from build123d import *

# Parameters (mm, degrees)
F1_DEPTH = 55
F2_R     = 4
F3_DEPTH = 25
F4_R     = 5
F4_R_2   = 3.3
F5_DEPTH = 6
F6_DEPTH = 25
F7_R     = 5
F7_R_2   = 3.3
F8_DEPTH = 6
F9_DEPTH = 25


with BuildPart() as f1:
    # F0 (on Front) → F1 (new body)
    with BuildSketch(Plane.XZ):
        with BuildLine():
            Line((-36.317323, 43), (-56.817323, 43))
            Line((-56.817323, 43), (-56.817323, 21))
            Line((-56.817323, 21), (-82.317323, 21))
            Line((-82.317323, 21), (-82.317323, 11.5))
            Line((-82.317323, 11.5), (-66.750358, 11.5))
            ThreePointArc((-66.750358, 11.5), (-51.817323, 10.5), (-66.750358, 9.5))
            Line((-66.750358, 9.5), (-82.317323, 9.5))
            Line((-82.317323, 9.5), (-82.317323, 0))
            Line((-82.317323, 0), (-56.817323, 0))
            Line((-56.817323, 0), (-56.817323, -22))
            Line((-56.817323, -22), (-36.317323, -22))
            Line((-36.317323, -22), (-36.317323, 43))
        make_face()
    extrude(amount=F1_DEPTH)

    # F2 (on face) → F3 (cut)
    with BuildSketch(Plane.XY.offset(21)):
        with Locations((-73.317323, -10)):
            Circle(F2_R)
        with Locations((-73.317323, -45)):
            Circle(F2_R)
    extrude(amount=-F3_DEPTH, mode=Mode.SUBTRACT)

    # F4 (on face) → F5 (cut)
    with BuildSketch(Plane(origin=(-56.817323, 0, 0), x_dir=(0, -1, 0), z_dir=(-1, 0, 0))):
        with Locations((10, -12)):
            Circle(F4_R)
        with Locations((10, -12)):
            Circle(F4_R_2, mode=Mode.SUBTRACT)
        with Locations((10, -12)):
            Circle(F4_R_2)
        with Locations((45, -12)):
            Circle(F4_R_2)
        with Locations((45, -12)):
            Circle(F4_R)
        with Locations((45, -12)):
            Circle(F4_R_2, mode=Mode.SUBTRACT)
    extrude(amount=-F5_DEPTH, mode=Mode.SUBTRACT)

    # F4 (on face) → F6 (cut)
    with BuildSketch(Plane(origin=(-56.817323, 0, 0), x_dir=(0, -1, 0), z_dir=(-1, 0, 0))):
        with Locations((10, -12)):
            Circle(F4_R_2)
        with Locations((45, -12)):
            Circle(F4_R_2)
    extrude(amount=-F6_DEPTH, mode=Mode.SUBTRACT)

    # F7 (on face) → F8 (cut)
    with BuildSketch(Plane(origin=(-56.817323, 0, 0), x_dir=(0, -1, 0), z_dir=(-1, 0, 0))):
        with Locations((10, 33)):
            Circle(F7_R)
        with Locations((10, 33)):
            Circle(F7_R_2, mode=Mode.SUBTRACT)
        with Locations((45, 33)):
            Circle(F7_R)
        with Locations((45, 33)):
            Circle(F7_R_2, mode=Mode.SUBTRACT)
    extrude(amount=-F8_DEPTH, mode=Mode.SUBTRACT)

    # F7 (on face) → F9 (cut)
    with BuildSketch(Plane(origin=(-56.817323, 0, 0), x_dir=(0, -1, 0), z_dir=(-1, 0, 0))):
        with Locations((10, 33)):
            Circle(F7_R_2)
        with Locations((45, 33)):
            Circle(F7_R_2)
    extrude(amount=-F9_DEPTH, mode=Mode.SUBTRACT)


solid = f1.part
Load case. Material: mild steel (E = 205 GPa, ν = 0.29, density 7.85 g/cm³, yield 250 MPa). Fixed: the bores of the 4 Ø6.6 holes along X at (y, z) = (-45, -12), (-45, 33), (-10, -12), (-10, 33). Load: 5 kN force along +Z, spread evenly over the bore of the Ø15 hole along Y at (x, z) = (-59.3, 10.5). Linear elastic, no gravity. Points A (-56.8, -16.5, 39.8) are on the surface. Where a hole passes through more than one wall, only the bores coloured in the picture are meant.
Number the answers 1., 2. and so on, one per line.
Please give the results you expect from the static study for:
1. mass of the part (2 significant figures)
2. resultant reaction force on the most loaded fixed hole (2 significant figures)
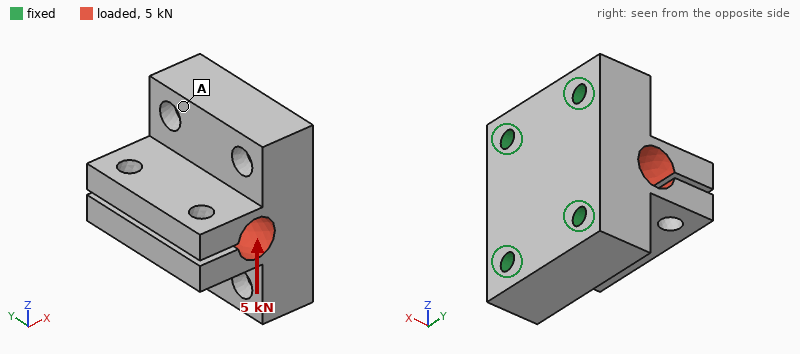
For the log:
1. 670 g
2. 1.5 kN
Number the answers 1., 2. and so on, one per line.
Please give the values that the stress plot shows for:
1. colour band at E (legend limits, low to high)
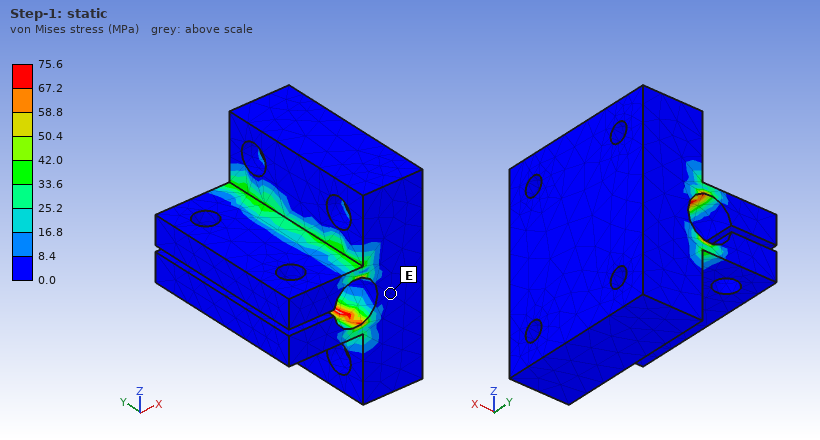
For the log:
1. 0.0 to 8.4 MPa
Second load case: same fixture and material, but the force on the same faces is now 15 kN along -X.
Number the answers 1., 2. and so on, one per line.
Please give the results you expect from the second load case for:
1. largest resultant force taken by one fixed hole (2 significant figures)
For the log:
1. 3.8 kN
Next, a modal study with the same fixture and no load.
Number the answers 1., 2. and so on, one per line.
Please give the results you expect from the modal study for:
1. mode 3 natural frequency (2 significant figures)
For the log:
1. 7100 Hz
